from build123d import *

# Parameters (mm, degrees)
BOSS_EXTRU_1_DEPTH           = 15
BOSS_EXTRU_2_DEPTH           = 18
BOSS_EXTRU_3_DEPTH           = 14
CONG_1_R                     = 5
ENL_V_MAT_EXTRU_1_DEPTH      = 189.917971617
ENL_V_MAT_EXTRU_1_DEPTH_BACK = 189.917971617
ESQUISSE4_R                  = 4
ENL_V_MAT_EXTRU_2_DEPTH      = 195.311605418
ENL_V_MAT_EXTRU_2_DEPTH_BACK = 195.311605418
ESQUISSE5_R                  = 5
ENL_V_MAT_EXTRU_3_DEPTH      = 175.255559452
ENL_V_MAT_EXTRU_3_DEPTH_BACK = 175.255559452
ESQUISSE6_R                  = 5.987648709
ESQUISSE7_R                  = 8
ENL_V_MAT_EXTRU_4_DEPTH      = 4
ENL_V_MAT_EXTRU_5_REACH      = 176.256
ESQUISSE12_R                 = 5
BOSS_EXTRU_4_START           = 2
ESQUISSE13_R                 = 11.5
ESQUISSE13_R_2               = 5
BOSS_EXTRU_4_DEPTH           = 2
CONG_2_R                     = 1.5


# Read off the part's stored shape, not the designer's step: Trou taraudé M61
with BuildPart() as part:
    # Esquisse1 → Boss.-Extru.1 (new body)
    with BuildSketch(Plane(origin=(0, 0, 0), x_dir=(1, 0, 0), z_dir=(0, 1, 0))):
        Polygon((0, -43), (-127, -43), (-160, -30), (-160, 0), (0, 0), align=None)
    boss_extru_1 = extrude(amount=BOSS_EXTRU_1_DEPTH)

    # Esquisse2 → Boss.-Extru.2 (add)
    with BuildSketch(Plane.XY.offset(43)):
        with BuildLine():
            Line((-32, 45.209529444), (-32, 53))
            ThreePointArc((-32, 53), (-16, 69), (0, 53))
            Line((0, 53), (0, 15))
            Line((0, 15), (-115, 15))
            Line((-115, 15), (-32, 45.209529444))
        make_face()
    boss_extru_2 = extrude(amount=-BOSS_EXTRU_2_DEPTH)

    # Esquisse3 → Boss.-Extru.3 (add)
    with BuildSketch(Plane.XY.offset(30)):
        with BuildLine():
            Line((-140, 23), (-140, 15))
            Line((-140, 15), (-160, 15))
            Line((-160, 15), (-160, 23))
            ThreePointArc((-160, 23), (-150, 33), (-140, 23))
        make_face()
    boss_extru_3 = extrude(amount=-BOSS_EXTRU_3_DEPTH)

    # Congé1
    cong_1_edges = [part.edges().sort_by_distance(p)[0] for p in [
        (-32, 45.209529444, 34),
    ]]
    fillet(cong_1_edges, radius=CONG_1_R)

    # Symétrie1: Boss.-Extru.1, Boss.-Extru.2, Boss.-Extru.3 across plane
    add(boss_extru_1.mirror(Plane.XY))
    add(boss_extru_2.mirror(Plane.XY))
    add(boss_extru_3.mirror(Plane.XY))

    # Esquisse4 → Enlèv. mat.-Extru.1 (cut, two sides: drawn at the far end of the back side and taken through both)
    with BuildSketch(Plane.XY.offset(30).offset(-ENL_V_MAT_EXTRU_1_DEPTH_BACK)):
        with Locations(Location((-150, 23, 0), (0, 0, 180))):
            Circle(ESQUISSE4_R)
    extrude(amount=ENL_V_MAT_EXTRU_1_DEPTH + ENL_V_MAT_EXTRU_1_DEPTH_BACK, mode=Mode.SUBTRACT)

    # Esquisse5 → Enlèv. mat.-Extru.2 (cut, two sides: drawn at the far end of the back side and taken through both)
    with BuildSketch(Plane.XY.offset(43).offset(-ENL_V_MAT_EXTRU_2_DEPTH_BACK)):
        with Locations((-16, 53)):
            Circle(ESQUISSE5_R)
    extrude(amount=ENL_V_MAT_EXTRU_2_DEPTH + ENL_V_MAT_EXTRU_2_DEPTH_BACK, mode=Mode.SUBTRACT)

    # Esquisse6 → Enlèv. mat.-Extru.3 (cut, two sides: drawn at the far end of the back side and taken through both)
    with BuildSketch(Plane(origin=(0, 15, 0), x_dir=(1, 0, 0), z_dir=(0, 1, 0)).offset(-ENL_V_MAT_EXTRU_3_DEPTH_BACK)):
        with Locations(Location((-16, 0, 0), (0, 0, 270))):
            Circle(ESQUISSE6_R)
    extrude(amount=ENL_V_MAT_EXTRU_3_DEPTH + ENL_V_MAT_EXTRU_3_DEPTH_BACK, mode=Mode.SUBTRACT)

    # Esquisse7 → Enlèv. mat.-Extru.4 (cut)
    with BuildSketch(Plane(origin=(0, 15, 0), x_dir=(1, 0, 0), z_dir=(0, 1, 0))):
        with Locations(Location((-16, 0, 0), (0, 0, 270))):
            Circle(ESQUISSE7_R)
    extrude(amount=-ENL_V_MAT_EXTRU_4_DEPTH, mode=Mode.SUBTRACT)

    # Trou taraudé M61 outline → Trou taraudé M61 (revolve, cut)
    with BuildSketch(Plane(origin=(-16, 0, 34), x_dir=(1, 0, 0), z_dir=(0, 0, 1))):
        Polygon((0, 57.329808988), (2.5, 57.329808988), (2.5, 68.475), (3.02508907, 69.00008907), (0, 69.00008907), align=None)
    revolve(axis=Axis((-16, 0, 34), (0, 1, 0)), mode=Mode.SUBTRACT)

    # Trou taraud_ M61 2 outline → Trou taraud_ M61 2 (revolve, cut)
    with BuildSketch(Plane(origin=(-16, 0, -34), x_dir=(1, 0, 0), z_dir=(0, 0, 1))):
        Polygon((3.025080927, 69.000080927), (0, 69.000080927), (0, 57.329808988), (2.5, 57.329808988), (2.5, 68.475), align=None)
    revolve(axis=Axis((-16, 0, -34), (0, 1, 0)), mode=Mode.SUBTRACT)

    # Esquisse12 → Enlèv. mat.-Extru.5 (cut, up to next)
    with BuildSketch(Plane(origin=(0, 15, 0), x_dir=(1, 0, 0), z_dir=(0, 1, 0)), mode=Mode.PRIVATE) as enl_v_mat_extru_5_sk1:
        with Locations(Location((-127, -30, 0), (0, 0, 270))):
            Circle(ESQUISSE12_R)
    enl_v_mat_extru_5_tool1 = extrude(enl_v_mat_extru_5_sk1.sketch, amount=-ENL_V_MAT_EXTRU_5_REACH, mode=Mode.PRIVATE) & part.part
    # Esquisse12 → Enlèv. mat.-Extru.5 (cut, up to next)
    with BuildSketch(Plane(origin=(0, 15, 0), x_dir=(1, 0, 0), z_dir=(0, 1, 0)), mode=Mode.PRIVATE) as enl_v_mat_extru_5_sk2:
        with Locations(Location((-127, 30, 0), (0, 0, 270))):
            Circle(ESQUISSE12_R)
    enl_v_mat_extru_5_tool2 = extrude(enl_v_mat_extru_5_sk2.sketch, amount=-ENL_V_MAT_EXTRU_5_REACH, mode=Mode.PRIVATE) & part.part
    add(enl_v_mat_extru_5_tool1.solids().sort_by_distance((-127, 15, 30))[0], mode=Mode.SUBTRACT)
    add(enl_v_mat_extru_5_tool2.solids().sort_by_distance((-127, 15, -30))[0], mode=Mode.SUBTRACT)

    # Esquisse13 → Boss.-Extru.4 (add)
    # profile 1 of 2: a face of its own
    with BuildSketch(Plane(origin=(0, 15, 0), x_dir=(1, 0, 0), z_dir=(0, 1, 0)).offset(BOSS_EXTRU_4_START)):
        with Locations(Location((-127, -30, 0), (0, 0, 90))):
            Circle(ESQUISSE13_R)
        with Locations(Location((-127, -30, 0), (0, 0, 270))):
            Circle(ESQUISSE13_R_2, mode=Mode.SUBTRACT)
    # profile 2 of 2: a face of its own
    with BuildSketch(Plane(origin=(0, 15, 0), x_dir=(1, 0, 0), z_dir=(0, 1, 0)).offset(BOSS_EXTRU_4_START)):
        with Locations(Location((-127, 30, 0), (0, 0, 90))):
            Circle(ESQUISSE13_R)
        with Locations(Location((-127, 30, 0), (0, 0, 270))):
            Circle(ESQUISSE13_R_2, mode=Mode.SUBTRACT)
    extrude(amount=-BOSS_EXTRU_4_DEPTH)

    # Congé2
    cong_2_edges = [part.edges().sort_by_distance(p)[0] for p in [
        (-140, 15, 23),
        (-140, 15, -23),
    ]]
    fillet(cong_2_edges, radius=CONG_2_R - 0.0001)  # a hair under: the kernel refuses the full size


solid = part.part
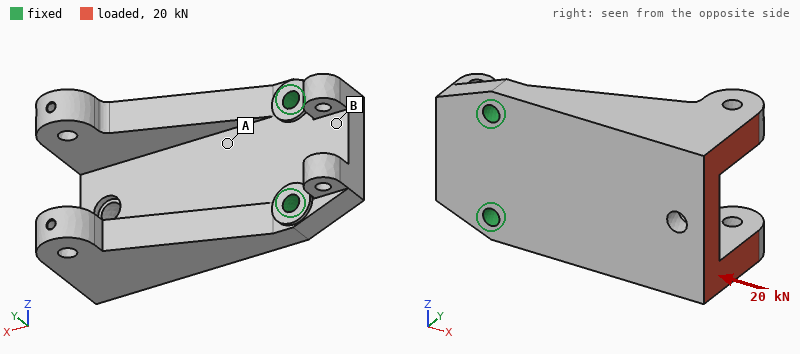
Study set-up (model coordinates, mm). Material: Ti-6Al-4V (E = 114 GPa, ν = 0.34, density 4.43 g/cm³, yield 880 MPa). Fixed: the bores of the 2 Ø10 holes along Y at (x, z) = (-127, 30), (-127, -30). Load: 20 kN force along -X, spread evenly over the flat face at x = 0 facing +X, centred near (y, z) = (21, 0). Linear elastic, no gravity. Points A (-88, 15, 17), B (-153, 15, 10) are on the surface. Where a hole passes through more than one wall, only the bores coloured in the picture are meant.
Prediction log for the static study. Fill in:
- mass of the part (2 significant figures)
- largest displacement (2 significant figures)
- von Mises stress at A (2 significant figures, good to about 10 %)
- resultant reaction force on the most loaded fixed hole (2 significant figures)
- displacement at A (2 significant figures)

1.3 kg
0.39 mm
37 MPa
10 kN
0.068 mm
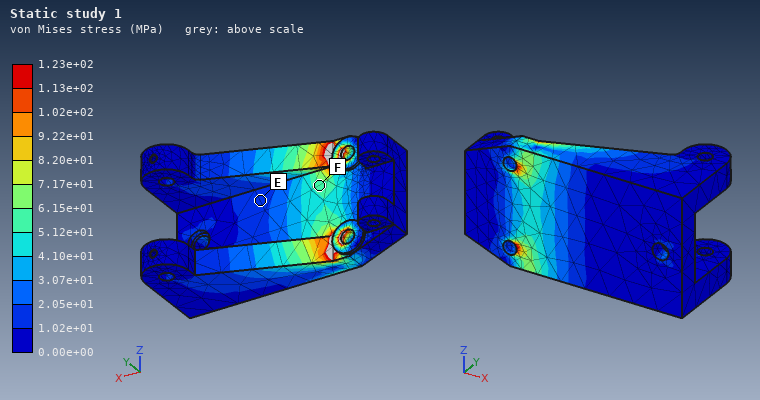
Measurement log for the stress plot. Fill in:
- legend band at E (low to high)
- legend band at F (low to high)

1.02e+01 to 2.05e+01 MPa
5.12e+01 to 6.15e+01 MPa
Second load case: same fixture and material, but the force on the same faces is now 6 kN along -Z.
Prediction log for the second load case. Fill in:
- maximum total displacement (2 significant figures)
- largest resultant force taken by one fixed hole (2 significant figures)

0.13 mm
12 kN
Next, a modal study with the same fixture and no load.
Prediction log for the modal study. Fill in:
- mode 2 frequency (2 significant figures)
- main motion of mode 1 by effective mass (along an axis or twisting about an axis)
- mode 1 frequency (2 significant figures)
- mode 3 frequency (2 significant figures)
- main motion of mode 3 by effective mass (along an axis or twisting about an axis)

1400 Hz
along Y
610 Hz
2500 Hz
along Z
